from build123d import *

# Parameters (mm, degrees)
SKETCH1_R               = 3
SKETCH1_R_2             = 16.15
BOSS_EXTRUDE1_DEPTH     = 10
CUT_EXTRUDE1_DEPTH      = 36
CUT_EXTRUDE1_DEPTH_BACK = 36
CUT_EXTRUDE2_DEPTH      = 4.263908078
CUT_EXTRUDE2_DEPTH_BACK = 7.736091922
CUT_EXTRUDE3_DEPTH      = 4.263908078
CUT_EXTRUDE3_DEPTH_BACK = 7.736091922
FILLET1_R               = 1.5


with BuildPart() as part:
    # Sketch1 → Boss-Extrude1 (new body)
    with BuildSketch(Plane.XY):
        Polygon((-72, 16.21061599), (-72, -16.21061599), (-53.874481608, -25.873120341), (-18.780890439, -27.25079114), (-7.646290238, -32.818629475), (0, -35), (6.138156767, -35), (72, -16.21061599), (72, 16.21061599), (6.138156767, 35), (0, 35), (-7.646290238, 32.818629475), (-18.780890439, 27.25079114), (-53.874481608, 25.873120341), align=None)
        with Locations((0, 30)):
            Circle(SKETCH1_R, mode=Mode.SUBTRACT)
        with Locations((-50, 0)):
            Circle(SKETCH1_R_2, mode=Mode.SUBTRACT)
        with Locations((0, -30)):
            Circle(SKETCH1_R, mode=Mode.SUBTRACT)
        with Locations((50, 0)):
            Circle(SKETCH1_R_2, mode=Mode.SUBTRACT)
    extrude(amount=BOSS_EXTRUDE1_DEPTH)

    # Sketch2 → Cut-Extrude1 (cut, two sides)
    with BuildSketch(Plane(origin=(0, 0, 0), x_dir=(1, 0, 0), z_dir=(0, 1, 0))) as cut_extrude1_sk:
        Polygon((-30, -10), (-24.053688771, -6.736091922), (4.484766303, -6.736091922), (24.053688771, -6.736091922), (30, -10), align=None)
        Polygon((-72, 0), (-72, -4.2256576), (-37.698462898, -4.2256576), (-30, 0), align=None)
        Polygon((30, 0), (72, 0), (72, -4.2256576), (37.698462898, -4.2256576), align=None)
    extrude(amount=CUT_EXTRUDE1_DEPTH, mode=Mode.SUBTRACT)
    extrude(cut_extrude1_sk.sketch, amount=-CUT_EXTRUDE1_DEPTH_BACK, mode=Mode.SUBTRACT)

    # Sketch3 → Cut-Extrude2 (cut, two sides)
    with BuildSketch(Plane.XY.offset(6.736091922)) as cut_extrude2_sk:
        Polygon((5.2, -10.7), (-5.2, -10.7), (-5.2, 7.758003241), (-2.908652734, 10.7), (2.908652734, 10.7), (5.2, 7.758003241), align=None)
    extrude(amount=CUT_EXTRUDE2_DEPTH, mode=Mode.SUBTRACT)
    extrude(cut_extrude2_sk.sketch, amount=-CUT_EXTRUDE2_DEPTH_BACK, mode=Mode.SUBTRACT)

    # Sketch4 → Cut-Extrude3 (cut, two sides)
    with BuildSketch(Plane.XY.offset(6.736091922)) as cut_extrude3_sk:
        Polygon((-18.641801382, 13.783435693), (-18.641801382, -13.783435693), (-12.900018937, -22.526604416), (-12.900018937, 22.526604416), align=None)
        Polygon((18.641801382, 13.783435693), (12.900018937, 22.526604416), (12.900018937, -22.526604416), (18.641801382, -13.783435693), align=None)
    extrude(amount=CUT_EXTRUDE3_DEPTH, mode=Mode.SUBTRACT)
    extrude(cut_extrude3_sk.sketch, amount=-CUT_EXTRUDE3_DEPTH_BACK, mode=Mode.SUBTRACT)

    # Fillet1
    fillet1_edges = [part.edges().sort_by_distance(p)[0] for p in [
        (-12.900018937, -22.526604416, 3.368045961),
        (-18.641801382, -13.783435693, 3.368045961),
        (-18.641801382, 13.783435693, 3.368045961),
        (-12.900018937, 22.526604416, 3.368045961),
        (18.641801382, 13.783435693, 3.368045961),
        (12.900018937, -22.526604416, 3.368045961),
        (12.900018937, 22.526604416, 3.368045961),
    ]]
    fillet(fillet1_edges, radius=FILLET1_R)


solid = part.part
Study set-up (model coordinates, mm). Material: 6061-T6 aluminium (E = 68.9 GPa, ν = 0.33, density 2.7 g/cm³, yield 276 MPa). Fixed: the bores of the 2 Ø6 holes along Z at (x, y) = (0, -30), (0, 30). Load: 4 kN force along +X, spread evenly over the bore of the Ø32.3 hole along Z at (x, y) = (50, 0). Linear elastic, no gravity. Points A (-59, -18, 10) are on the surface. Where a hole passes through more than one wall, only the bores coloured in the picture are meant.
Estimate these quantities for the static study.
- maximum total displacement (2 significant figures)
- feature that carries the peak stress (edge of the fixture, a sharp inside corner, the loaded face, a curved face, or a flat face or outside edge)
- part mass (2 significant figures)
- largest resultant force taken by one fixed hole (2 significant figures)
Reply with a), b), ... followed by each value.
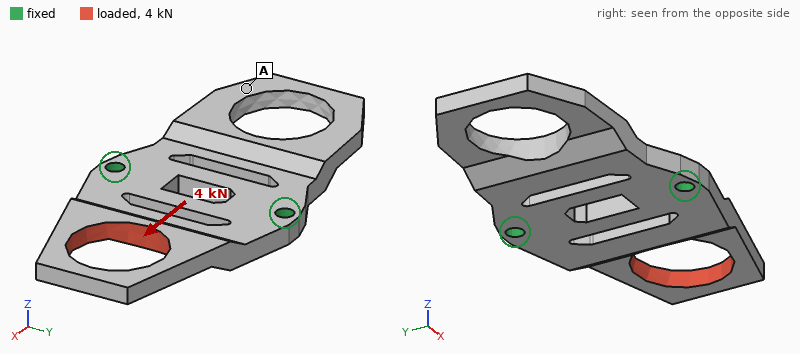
a) 0.42 mm
b) a curved face
c) 98 g
d) 2.1 kN
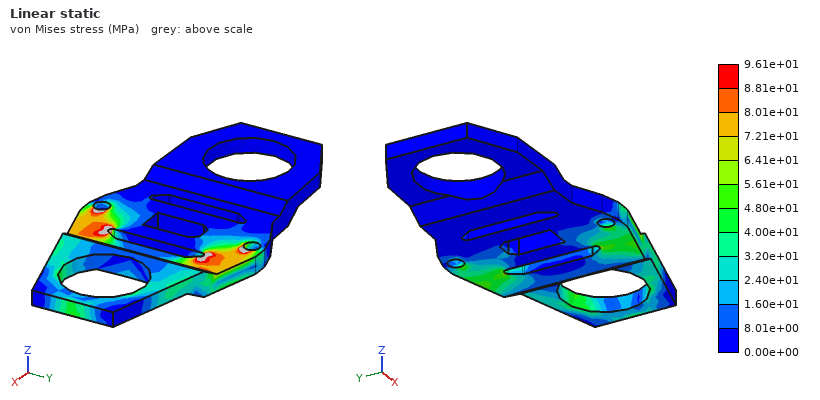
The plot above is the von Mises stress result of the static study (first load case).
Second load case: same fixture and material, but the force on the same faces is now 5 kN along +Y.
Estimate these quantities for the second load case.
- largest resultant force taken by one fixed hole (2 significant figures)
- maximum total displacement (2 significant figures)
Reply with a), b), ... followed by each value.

a) 4.5 kN
b) 0.22 mm
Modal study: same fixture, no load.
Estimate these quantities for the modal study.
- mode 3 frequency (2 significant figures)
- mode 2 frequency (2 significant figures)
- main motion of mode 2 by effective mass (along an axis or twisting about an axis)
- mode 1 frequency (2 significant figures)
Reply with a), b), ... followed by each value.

a) 3600 Hz
b) 1300 Hz
c) along Z
d) 1100 Hz
